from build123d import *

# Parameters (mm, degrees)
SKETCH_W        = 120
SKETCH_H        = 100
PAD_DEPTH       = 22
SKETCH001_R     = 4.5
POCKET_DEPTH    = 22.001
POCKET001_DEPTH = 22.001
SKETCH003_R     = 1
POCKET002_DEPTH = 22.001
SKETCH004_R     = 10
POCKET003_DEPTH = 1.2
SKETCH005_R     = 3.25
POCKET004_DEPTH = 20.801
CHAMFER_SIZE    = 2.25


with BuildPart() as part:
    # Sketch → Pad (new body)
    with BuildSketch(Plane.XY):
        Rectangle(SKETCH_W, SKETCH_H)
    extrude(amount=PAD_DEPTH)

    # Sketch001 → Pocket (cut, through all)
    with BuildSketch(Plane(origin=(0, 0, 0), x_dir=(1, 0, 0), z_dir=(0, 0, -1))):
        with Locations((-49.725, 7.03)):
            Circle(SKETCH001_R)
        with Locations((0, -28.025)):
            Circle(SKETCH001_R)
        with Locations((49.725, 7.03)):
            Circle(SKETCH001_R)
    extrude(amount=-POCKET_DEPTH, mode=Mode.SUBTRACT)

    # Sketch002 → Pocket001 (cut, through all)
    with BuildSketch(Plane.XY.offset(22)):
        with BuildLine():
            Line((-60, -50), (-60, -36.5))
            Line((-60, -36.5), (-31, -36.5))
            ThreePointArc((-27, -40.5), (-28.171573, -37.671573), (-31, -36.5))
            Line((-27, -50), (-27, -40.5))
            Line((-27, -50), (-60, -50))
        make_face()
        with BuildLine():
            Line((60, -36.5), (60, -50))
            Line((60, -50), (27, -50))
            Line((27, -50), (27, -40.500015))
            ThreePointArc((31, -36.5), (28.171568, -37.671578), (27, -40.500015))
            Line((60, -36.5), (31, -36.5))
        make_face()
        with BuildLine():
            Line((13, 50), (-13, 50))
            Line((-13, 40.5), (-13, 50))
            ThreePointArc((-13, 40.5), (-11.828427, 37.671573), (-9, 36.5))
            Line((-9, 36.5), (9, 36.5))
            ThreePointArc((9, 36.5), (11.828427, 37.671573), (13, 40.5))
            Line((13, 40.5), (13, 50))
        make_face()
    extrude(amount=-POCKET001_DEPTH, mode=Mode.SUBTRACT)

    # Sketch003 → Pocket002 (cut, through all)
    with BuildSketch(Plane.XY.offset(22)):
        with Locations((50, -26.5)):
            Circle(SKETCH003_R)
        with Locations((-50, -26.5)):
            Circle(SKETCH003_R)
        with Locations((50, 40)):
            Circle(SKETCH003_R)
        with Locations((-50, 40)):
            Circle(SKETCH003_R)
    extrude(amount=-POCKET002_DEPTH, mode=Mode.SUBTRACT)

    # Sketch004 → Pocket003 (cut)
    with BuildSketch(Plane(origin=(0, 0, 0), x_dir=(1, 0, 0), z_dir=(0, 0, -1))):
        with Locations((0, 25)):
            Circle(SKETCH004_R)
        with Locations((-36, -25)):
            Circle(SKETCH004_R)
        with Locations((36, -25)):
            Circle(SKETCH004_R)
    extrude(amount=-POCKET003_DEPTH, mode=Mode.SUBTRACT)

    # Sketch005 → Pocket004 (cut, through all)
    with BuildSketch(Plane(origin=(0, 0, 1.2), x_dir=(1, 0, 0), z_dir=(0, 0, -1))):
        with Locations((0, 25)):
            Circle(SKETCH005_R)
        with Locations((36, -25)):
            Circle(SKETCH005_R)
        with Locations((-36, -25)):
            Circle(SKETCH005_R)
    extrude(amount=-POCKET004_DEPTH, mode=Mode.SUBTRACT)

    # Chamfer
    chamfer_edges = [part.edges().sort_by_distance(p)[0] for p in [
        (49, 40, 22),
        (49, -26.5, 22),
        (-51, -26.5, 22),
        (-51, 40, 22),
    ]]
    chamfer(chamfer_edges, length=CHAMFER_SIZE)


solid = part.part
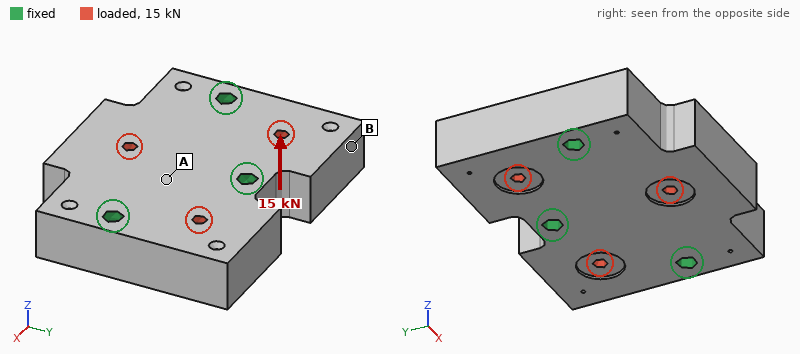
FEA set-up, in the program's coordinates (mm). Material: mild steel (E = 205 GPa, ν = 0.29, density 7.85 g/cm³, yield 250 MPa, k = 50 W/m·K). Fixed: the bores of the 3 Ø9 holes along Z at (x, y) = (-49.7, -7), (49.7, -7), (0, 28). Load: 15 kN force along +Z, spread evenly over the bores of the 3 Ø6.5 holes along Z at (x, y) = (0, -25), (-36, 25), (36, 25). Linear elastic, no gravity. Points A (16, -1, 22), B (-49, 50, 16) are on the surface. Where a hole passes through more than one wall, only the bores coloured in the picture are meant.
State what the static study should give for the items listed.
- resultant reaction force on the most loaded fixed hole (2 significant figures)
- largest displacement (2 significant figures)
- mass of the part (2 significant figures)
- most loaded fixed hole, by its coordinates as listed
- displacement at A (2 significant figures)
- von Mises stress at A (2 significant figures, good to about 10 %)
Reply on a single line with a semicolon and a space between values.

6.1 kN; 7.5 µm; 1.8 kg; (0, 28); 2.4 µm; 11 MPa
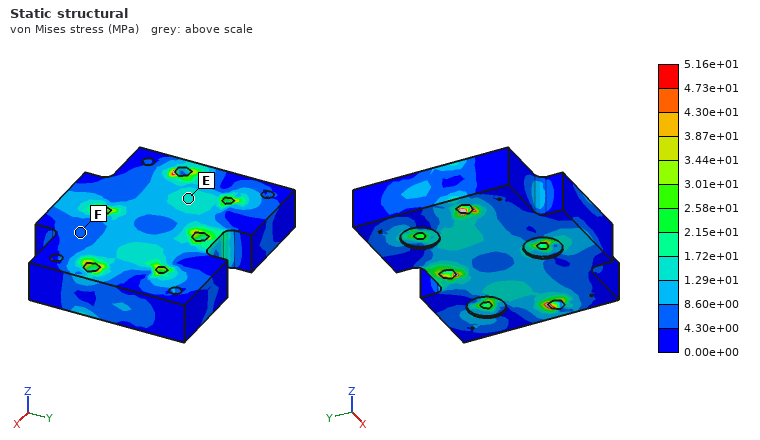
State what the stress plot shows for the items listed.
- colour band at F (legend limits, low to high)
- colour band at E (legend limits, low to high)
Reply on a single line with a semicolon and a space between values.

4.30e+00 to 8.60e+00 MPa; 1.29e+01 to 1.72e+01 MPa
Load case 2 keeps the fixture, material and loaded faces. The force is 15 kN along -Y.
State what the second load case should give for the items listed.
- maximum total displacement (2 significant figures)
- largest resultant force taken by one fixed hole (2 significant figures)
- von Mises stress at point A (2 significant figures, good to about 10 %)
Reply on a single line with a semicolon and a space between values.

1.9 µm; 5.3 kN; 2.9 MPa
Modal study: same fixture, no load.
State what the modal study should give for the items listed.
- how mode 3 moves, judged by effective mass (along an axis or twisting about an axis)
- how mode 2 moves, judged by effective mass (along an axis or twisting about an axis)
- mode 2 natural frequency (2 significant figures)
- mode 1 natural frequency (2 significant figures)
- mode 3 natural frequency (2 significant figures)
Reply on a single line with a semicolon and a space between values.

along Z; twisting about Y; 7600 Hz; 5900 Hz; 8000 Hz
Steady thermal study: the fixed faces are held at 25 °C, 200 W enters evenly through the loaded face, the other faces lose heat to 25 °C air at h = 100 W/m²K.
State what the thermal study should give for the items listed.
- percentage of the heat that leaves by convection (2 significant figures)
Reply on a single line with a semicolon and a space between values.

27 %
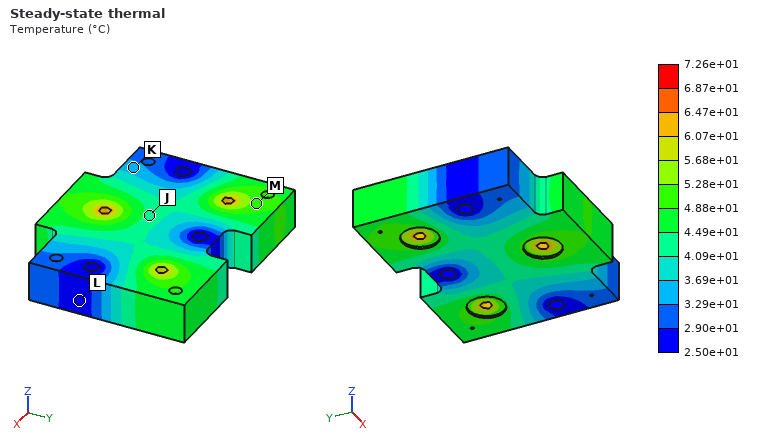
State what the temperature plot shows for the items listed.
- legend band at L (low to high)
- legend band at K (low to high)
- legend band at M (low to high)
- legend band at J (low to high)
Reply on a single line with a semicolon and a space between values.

2.50e+01 to 2.90e+01 °C; 3.29e+01 to 3.69e+01 °C; 4.88e+01 to 5.28e+01 °C; 4.09e+01 to 4.49e+01 °C
